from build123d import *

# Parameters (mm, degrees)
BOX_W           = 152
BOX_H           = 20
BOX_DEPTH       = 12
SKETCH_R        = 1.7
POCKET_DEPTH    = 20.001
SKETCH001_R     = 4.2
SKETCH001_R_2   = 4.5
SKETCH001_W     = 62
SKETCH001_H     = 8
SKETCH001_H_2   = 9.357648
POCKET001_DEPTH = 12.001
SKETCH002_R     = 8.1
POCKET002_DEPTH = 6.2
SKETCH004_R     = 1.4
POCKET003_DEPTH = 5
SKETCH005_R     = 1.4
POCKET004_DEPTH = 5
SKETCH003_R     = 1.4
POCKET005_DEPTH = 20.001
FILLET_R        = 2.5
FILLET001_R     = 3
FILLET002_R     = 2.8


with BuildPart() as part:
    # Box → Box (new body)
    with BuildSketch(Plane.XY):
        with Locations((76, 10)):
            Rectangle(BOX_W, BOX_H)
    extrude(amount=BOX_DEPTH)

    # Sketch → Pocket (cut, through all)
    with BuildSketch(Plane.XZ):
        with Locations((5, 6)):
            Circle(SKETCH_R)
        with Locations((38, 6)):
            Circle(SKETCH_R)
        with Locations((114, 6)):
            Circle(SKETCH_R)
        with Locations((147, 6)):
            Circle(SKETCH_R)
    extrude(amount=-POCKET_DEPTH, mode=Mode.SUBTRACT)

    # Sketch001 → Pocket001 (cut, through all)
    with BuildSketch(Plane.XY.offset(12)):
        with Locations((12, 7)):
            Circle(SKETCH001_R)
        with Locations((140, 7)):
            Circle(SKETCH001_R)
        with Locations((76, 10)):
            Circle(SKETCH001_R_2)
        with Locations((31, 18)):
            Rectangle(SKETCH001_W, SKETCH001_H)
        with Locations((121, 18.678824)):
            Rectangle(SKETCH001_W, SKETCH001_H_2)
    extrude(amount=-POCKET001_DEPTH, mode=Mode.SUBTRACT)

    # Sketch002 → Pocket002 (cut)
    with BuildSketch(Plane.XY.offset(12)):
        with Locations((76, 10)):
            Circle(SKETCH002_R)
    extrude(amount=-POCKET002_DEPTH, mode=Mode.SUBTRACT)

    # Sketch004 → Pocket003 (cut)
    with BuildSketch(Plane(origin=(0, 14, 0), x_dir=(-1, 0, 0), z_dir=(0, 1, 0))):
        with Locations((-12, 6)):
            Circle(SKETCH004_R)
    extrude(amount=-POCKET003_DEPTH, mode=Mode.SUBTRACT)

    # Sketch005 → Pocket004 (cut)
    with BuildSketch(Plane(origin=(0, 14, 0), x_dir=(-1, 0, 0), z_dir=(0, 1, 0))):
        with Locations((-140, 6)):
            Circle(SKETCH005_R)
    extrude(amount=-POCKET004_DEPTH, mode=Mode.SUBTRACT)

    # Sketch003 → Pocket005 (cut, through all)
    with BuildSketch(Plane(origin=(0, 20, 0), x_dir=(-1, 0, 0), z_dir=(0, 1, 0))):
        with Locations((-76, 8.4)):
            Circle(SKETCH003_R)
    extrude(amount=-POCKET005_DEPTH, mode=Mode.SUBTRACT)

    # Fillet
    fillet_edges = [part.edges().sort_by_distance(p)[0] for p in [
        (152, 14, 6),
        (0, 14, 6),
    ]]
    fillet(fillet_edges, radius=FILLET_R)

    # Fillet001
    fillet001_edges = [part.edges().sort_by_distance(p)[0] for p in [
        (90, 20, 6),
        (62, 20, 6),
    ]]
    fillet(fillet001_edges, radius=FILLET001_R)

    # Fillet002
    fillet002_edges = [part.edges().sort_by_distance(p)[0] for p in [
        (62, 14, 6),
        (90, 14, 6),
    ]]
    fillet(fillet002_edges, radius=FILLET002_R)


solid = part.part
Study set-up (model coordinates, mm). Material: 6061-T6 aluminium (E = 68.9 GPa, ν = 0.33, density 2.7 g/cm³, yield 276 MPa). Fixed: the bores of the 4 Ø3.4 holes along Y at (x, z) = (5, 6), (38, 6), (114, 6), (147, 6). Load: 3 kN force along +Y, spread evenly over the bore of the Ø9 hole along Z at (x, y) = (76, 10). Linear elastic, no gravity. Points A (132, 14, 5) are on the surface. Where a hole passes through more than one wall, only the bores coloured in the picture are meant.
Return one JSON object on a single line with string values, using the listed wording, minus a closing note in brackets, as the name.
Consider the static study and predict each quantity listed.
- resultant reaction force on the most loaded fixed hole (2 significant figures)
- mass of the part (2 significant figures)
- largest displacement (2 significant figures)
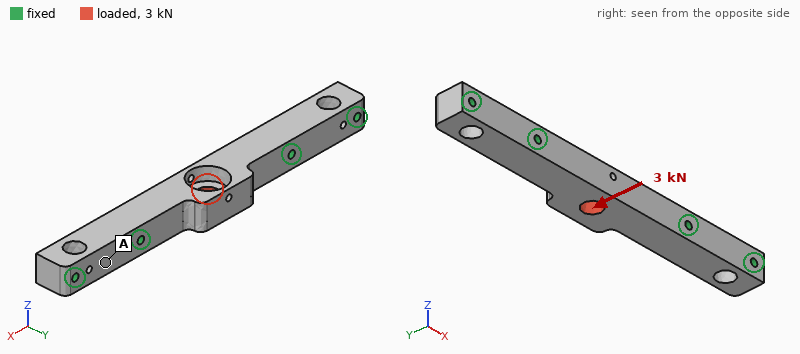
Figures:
{"resultant reaction force on the most loaded fixed hole": "1.6 kN", "mass of the part": "65 g", "largest displacement": "52 µm"}
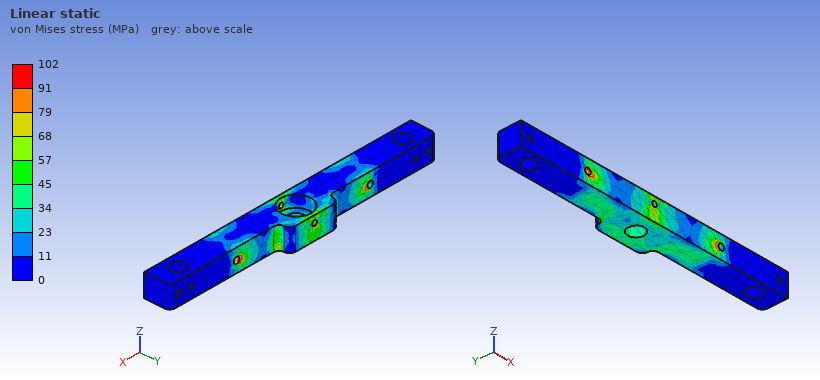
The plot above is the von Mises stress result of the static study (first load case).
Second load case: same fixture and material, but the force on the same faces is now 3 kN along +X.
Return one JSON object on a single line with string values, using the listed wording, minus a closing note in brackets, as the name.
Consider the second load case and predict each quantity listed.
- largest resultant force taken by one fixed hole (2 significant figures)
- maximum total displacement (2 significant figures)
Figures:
{"largest resultant force taken by one fixed hole": "1.5 kN", "maximum total displacement": "7.8 µm"}
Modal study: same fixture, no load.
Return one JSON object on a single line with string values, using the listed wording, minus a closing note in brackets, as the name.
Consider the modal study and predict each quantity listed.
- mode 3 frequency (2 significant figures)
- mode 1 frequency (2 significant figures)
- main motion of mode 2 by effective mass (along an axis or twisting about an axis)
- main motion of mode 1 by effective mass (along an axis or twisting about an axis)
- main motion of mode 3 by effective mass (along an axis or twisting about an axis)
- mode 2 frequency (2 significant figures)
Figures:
{"mode 3 frequency": "15 kHz", "mode 1 frequency": "7100 Hz", "main motion of mode 2 by effective mass": "along Y", "main motion of mode 1 by effective mass": "along Z", "main motion of mode 3 by effective mass": "twisting about X", "mode 2 frequency": "11 kHz"}
